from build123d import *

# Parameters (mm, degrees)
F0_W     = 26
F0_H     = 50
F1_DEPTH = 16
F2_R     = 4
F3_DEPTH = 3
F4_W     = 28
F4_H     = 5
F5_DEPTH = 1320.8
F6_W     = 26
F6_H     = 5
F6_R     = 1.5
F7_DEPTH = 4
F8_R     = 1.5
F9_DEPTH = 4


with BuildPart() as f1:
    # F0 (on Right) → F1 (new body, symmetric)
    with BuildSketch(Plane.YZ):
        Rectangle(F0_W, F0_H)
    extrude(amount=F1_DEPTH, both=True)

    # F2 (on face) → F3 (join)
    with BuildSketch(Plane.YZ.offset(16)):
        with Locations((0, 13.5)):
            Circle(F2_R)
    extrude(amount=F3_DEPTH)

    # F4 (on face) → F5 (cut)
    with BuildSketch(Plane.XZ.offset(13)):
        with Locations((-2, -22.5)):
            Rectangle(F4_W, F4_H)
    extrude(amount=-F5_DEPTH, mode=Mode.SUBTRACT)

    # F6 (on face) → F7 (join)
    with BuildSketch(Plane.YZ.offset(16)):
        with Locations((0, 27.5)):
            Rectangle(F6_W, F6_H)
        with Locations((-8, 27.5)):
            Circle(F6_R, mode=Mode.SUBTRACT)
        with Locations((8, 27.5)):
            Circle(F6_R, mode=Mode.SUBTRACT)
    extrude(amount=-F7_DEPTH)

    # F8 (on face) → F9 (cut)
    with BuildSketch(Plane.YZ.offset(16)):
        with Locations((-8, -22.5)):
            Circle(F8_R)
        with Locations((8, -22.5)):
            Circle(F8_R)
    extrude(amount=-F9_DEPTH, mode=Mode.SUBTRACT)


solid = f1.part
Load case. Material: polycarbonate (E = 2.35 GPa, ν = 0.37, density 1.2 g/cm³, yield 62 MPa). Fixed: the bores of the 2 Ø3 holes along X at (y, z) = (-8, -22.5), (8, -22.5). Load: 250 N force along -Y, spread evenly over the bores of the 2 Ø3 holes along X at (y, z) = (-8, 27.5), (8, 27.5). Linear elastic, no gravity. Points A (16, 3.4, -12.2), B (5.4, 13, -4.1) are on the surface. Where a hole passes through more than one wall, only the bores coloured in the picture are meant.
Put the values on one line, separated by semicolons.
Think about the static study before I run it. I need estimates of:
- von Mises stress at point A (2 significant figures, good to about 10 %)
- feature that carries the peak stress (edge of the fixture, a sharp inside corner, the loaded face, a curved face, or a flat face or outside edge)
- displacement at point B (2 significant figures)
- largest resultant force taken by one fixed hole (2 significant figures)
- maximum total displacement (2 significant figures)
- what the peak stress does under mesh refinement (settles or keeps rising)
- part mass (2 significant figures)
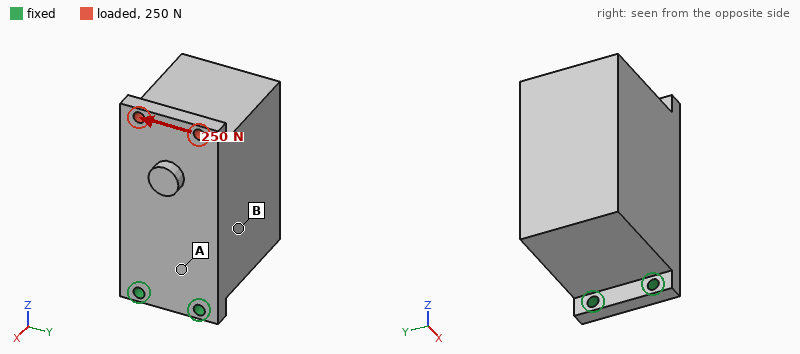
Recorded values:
8.9 MPa; edge of the fixture; 0.22 mm; 720 N; 0.70 mm; keeps rising; 46 g
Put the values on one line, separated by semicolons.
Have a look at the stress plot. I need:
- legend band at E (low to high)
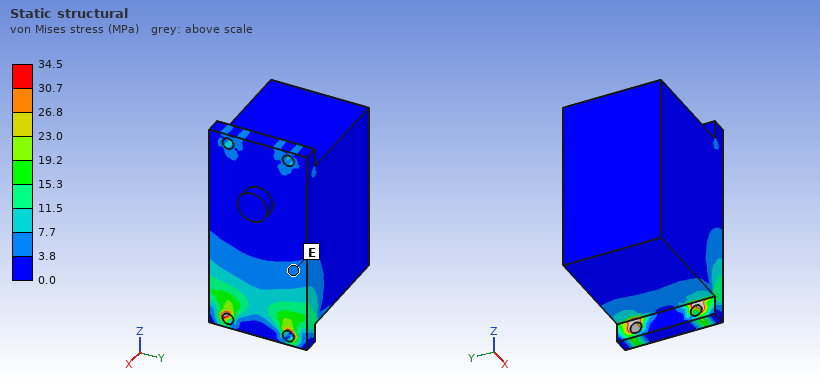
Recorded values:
3.8 to 7.7 MPa
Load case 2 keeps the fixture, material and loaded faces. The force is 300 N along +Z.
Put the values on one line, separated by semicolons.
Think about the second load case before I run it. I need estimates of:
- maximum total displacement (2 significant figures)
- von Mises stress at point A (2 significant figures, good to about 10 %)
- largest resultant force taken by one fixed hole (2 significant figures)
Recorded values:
0.13 mm; 2.1 MPa; 150 N
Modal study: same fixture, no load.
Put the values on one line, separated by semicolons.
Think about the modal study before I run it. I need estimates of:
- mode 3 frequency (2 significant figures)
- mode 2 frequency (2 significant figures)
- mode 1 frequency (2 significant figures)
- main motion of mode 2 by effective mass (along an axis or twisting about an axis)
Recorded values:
1300 Hz; 830 Hz; 190 Hz; along Y
